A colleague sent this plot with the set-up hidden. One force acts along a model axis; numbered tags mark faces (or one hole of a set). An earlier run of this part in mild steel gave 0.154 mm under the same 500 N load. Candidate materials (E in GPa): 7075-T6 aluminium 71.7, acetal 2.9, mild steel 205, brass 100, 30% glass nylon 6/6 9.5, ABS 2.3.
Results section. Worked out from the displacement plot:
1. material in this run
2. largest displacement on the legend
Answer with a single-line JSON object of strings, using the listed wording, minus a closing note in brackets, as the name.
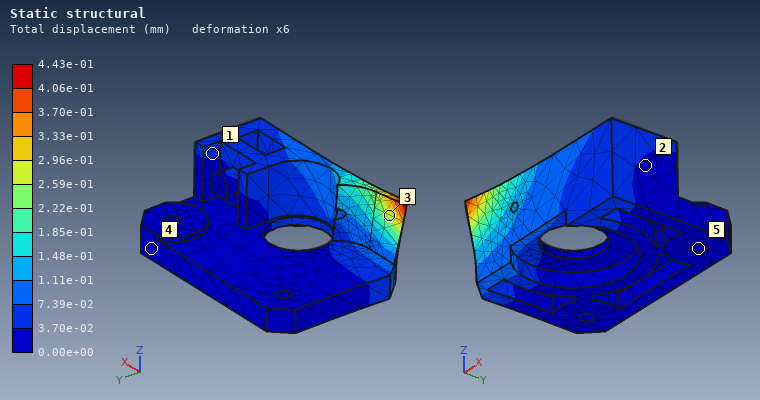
{"material in this run": "7075-T6 aluminium", "largest displacement on the legend": "4.43e-01 mm"}
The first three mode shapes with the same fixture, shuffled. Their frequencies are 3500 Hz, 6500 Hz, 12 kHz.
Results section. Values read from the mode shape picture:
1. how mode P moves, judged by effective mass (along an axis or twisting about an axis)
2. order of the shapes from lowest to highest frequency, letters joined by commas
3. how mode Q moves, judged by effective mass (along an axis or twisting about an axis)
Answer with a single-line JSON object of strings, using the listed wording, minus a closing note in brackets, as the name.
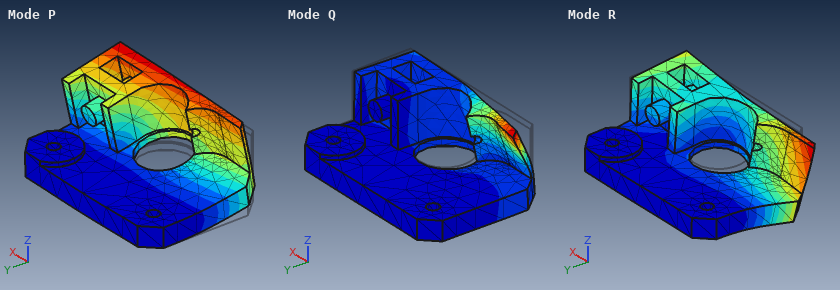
{"how mode P moves, judged by effective mass": "along Z", "order of the shapes from lowest to highest frequency, letters joined by commas": "P, R, Q", "how mode Q moves, judged by effective mass": "along X"}
